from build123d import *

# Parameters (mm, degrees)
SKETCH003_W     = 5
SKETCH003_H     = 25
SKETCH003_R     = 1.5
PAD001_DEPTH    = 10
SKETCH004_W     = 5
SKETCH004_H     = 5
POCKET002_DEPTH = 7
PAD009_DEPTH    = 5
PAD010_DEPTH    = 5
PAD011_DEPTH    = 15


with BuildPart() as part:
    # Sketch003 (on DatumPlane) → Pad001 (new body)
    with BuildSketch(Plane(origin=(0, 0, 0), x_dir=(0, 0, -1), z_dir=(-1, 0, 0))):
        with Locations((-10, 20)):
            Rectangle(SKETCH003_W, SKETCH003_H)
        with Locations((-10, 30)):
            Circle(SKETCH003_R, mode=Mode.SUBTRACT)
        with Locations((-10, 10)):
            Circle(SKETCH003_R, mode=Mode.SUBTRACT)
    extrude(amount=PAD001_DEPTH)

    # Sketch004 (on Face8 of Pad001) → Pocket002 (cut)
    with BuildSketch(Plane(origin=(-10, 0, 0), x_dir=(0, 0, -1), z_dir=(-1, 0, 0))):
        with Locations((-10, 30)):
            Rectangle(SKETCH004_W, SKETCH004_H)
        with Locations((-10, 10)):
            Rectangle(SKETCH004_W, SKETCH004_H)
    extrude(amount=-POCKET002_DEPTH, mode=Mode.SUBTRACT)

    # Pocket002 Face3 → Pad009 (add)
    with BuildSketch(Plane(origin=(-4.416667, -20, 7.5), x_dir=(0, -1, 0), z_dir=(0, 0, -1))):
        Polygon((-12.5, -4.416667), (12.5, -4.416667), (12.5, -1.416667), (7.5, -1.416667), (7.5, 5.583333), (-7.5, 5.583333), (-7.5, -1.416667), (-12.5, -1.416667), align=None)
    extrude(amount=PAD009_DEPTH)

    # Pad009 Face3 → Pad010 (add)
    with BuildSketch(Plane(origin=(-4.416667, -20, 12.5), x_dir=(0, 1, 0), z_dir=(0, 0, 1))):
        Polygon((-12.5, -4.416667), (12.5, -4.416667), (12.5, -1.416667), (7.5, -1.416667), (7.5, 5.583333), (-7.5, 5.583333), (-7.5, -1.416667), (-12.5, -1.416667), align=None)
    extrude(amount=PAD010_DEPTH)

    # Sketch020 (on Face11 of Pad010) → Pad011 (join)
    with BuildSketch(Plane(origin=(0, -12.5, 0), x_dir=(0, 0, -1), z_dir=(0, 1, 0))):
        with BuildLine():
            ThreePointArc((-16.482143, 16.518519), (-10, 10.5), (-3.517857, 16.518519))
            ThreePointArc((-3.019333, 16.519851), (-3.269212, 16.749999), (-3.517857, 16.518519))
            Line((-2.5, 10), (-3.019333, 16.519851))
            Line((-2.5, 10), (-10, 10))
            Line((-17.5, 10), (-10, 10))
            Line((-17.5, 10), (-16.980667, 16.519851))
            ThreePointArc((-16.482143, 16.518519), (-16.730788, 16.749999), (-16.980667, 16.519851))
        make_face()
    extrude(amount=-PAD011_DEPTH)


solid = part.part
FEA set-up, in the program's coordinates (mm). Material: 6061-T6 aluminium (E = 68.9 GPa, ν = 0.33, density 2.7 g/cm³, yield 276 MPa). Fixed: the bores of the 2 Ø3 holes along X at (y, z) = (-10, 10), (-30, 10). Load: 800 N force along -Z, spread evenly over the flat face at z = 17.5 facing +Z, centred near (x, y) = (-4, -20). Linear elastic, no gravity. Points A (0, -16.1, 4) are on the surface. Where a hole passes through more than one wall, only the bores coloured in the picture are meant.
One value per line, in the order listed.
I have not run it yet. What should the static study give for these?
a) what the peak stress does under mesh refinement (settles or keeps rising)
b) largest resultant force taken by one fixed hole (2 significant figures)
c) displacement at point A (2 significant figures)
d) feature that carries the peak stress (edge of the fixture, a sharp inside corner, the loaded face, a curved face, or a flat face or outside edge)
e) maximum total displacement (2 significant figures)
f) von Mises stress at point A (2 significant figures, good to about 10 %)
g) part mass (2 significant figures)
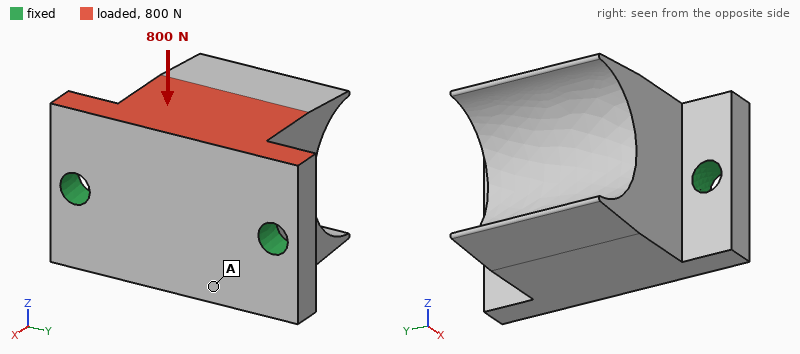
keeps rising
400 N
7.0 µm
edge of the fixture
22 µm
13 MPa
8.6 g
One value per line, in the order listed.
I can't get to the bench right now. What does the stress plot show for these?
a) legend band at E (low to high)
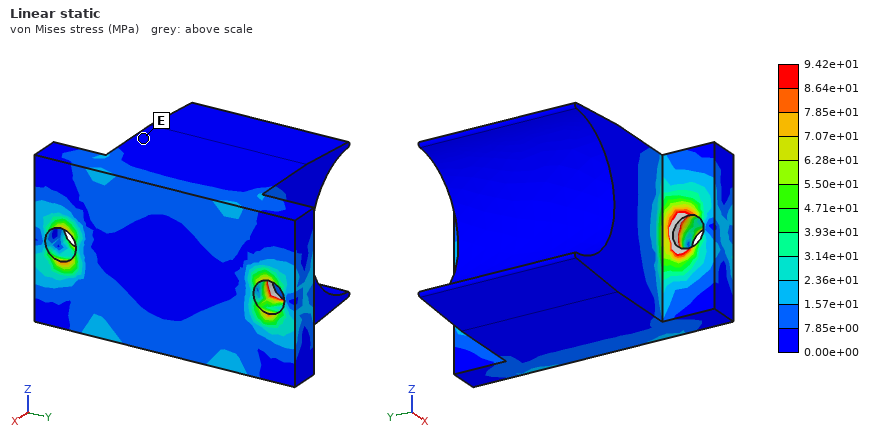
0.00e+00 to 7.85e+00 MPa
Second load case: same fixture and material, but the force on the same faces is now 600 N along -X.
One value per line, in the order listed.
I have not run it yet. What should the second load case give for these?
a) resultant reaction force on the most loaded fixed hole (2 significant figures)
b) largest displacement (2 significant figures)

320 N
38 µm
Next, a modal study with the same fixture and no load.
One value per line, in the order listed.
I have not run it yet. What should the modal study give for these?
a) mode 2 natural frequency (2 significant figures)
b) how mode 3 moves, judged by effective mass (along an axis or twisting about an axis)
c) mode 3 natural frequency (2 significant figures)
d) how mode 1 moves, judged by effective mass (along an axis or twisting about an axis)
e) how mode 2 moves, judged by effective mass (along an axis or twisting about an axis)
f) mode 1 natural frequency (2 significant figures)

28 kHz
along Y
30 kHz
along Z
along X
10 kHz
